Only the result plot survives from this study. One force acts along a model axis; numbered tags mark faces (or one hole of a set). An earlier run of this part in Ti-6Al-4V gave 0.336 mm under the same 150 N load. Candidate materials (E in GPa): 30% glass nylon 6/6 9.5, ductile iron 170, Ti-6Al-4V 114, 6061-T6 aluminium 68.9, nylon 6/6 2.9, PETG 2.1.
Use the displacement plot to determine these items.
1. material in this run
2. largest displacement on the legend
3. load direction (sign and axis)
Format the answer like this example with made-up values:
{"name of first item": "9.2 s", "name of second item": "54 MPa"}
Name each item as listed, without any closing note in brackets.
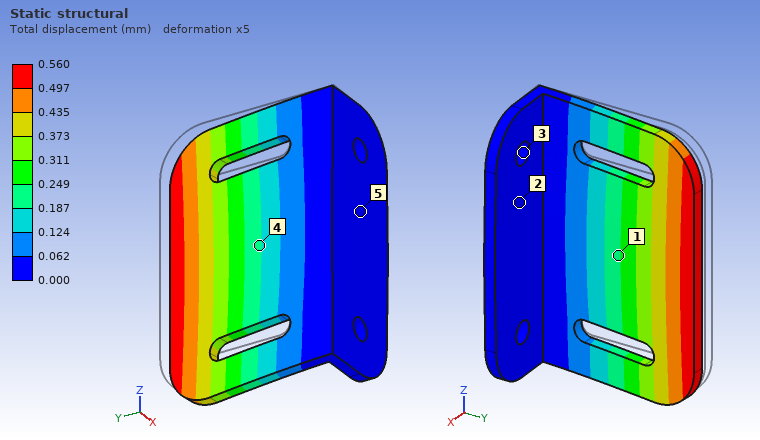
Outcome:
{"material in this run": "6061-T6 aluminium", "largest displacement on the legend": "0.560 mm", "load direction": "+X"}
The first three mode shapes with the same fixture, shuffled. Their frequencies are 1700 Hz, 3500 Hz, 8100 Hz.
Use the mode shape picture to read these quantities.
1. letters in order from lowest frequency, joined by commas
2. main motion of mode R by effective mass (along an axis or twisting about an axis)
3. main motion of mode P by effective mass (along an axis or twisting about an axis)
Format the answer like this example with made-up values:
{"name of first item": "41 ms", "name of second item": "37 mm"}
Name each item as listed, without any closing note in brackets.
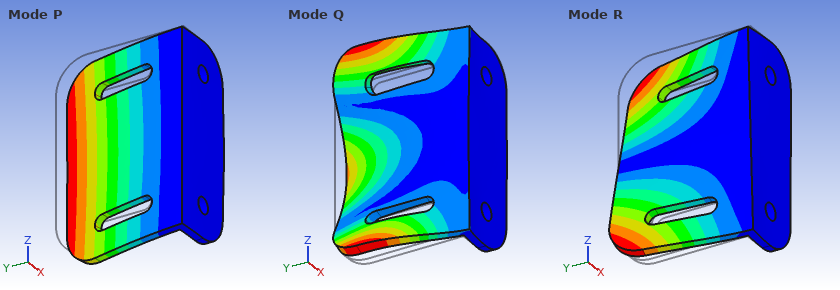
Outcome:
{"letters in order from lowest frequency, joined by commas": "P, R, Q", "main motion of mode R by effective mass": "twisting about Y", "main motion of mode P by effective mass": "along X"}
